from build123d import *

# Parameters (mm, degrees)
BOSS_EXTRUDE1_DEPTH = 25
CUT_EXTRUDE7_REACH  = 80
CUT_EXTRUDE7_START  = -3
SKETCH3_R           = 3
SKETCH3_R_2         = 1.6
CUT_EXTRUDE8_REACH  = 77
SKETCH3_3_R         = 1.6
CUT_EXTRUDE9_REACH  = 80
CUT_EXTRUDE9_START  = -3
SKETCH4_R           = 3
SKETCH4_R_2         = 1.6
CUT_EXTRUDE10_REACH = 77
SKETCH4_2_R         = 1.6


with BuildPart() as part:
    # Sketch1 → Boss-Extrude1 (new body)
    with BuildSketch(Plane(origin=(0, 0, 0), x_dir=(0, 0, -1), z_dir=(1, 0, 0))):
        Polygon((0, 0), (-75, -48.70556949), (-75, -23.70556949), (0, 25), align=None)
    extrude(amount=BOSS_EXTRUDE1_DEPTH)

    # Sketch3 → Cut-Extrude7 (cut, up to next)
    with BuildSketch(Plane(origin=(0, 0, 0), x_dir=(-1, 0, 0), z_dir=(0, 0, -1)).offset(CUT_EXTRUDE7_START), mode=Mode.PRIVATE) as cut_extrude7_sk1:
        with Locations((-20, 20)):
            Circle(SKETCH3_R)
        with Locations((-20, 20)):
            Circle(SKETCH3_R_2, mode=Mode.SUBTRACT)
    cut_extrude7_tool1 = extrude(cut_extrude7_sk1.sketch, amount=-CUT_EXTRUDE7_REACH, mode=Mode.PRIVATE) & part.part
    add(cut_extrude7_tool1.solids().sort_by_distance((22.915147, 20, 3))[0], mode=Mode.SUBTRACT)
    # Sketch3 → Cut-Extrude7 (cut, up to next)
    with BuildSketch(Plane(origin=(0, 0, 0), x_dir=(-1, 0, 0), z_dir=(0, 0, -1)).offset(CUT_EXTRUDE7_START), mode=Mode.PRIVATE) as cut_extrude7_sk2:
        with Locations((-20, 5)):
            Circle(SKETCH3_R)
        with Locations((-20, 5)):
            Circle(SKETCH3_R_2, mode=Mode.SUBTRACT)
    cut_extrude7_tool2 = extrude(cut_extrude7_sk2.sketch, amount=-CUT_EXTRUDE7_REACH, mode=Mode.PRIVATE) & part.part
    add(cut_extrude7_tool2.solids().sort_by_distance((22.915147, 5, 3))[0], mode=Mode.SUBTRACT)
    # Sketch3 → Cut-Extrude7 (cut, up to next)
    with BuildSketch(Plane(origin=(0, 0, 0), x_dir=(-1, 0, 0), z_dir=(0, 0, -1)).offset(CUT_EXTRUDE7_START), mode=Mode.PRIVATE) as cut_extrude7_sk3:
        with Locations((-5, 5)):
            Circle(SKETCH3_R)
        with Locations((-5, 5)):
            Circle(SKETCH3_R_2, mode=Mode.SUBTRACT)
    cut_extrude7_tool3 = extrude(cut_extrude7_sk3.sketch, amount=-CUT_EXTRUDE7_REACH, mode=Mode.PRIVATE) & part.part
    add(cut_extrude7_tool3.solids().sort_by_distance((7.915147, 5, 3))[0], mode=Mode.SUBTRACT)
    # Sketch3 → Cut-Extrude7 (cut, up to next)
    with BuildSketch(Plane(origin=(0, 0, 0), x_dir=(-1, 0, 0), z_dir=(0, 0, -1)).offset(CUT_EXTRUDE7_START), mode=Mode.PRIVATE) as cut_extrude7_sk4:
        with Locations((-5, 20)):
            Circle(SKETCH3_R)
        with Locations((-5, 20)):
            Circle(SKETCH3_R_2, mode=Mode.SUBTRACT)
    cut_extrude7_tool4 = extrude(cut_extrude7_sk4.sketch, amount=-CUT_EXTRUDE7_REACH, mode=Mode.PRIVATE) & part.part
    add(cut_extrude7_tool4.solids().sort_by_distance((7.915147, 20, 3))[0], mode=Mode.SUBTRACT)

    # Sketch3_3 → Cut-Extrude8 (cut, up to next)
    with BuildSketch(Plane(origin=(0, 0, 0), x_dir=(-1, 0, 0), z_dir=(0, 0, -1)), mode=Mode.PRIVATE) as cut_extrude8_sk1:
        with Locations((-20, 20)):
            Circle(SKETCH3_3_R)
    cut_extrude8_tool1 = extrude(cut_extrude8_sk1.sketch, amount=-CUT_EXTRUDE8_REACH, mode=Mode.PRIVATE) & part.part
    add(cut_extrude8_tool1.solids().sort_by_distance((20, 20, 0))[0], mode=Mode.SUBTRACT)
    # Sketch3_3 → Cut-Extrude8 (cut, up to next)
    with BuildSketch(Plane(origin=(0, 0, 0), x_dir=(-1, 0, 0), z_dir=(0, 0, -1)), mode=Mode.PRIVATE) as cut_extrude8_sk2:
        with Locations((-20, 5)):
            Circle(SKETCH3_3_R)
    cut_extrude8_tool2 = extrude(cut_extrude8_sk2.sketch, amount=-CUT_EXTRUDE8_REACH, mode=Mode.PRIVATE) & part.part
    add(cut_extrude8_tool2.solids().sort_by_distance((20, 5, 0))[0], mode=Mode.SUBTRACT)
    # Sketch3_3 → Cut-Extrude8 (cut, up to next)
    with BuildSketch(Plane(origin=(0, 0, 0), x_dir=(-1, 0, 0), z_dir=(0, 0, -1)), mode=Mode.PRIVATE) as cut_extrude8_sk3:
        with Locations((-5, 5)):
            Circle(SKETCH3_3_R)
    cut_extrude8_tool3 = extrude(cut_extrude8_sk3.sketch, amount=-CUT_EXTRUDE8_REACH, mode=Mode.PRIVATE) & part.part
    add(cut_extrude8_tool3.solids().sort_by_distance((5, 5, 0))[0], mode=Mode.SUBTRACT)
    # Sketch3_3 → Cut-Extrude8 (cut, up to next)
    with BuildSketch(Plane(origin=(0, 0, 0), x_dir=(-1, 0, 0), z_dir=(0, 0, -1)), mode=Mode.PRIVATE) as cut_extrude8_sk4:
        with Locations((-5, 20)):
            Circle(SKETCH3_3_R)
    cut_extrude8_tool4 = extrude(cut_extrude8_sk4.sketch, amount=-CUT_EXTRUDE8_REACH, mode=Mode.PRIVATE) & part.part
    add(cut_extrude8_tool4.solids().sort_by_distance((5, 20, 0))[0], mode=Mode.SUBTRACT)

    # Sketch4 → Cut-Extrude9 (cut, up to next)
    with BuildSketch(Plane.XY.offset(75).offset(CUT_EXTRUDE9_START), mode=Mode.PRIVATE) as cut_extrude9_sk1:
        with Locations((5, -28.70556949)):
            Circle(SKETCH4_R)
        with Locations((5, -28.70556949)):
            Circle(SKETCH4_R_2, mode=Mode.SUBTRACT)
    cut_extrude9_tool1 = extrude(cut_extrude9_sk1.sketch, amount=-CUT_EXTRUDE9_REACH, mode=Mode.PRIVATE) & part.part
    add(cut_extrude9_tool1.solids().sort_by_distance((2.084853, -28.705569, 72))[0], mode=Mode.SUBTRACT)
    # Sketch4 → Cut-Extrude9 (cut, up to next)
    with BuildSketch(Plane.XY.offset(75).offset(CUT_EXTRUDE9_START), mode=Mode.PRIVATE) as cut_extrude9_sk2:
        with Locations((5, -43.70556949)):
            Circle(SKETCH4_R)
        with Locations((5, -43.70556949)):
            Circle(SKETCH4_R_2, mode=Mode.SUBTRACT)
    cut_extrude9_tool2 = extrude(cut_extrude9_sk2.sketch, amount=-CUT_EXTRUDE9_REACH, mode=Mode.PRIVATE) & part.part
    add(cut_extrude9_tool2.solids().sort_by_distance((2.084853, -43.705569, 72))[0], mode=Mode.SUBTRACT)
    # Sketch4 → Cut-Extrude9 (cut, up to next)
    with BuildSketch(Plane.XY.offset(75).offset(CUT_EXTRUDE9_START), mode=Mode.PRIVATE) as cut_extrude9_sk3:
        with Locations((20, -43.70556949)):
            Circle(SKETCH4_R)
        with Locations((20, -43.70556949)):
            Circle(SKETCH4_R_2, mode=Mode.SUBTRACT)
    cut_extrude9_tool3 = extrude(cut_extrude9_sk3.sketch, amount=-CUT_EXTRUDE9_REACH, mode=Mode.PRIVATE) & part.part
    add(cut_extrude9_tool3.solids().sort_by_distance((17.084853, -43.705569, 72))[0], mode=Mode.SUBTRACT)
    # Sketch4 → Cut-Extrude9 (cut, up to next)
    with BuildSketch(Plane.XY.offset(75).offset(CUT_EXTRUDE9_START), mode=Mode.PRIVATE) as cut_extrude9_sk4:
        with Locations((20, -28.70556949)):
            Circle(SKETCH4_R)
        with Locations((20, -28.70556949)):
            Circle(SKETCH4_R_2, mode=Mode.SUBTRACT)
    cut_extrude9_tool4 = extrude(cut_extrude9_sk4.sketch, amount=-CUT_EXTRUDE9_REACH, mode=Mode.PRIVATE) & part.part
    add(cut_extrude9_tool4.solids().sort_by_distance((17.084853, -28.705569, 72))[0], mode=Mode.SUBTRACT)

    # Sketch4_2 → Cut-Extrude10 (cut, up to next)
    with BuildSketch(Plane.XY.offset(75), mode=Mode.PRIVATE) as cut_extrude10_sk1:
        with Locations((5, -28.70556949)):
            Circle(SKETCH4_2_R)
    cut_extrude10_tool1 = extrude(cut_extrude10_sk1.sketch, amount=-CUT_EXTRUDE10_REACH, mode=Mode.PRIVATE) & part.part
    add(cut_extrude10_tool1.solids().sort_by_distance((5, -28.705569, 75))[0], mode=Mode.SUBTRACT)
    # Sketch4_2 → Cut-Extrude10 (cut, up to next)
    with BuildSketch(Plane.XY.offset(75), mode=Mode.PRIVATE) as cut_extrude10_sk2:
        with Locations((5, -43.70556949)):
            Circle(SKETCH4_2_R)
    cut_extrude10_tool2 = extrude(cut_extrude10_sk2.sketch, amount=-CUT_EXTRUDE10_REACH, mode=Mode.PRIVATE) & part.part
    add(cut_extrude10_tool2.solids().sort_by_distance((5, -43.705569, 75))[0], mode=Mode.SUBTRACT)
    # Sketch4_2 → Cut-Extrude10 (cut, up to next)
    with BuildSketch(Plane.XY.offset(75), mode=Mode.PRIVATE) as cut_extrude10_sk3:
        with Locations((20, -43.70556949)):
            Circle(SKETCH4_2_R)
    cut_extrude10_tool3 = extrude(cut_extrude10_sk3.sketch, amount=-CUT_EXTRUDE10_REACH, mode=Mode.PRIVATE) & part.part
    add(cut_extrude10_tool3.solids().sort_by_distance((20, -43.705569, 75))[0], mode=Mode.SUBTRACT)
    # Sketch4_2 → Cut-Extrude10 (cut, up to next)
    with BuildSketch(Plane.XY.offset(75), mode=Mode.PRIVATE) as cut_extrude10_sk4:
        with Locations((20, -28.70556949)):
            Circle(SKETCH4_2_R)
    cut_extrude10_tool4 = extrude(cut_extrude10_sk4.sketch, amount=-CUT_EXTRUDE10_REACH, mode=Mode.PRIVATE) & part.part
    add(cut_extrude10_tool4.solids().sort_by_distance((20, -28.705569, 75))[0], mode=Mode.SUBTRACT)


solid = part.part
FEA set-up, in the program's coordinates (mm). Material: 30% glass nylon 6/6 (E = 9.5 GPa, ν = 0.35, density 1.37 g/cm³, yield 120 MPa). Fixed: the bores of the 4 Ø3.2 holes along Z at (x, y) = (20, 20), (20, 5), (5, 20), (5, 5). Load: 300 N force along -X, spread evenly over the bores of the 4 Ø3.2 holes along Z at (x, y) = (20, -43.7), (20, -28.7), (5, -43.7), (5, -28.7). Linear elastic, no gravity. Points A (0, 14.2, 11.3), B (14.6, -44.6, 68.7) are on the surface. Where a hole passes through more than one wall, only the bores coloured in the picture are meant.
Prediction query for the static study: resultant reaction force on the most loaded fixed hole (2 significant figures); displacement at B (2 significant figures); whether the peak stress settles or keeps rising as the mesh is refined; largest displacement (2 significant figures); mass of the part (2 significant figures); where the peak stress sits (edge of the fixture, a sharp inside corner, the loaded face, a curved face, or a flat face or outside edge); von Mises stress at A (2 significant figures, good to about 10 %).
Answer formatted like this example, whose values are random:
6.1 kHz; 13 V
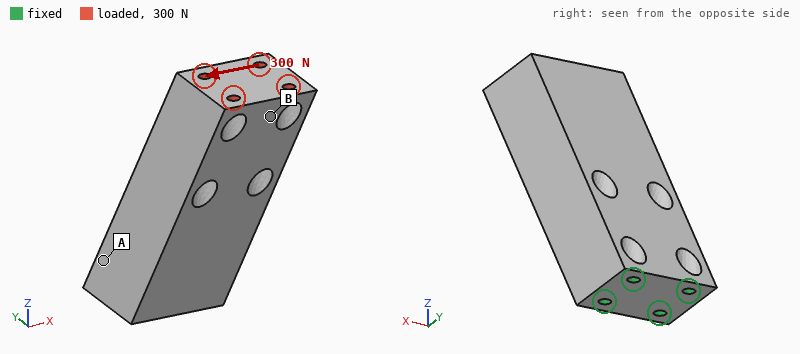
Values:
940 N; 0.46 mm; keeps rising; 0.52 mm; 59 g; edge of the fixture; 12 MPa
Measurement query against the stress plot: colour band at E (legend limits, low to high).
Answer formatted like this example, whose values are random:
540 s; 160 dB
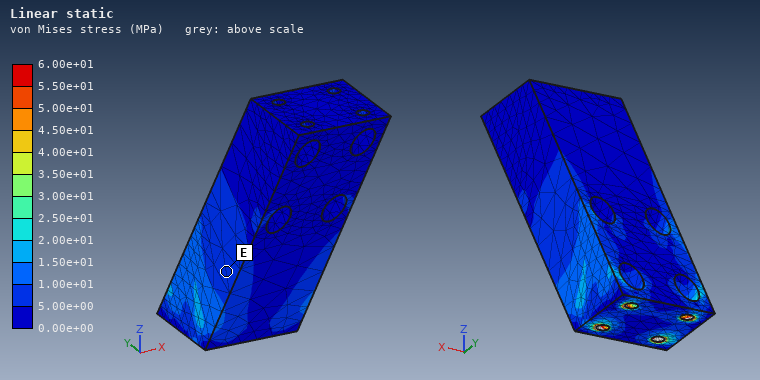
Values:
5.00e+00 to 1.00e+01 MPa
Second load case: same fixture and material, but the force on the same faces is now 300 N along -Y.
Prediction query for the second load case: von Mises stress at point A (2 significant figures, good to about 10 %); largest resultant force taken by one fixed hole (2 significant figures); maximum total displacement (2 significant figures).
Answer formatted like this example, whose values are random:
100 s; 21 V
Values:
11 MPa; 730 N; 0.62 mm
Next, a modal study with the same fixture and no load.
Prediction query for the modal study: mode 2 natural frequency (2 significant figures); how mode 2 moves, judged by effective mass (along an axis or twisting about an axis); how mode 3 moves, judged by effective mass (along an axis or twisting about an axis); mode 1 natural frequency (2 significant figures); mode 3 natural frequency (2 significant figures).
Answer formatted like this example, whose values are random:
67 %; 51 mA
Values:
990 Hz; along X; twisting about Z; 830 Hz; 3700 Hz
